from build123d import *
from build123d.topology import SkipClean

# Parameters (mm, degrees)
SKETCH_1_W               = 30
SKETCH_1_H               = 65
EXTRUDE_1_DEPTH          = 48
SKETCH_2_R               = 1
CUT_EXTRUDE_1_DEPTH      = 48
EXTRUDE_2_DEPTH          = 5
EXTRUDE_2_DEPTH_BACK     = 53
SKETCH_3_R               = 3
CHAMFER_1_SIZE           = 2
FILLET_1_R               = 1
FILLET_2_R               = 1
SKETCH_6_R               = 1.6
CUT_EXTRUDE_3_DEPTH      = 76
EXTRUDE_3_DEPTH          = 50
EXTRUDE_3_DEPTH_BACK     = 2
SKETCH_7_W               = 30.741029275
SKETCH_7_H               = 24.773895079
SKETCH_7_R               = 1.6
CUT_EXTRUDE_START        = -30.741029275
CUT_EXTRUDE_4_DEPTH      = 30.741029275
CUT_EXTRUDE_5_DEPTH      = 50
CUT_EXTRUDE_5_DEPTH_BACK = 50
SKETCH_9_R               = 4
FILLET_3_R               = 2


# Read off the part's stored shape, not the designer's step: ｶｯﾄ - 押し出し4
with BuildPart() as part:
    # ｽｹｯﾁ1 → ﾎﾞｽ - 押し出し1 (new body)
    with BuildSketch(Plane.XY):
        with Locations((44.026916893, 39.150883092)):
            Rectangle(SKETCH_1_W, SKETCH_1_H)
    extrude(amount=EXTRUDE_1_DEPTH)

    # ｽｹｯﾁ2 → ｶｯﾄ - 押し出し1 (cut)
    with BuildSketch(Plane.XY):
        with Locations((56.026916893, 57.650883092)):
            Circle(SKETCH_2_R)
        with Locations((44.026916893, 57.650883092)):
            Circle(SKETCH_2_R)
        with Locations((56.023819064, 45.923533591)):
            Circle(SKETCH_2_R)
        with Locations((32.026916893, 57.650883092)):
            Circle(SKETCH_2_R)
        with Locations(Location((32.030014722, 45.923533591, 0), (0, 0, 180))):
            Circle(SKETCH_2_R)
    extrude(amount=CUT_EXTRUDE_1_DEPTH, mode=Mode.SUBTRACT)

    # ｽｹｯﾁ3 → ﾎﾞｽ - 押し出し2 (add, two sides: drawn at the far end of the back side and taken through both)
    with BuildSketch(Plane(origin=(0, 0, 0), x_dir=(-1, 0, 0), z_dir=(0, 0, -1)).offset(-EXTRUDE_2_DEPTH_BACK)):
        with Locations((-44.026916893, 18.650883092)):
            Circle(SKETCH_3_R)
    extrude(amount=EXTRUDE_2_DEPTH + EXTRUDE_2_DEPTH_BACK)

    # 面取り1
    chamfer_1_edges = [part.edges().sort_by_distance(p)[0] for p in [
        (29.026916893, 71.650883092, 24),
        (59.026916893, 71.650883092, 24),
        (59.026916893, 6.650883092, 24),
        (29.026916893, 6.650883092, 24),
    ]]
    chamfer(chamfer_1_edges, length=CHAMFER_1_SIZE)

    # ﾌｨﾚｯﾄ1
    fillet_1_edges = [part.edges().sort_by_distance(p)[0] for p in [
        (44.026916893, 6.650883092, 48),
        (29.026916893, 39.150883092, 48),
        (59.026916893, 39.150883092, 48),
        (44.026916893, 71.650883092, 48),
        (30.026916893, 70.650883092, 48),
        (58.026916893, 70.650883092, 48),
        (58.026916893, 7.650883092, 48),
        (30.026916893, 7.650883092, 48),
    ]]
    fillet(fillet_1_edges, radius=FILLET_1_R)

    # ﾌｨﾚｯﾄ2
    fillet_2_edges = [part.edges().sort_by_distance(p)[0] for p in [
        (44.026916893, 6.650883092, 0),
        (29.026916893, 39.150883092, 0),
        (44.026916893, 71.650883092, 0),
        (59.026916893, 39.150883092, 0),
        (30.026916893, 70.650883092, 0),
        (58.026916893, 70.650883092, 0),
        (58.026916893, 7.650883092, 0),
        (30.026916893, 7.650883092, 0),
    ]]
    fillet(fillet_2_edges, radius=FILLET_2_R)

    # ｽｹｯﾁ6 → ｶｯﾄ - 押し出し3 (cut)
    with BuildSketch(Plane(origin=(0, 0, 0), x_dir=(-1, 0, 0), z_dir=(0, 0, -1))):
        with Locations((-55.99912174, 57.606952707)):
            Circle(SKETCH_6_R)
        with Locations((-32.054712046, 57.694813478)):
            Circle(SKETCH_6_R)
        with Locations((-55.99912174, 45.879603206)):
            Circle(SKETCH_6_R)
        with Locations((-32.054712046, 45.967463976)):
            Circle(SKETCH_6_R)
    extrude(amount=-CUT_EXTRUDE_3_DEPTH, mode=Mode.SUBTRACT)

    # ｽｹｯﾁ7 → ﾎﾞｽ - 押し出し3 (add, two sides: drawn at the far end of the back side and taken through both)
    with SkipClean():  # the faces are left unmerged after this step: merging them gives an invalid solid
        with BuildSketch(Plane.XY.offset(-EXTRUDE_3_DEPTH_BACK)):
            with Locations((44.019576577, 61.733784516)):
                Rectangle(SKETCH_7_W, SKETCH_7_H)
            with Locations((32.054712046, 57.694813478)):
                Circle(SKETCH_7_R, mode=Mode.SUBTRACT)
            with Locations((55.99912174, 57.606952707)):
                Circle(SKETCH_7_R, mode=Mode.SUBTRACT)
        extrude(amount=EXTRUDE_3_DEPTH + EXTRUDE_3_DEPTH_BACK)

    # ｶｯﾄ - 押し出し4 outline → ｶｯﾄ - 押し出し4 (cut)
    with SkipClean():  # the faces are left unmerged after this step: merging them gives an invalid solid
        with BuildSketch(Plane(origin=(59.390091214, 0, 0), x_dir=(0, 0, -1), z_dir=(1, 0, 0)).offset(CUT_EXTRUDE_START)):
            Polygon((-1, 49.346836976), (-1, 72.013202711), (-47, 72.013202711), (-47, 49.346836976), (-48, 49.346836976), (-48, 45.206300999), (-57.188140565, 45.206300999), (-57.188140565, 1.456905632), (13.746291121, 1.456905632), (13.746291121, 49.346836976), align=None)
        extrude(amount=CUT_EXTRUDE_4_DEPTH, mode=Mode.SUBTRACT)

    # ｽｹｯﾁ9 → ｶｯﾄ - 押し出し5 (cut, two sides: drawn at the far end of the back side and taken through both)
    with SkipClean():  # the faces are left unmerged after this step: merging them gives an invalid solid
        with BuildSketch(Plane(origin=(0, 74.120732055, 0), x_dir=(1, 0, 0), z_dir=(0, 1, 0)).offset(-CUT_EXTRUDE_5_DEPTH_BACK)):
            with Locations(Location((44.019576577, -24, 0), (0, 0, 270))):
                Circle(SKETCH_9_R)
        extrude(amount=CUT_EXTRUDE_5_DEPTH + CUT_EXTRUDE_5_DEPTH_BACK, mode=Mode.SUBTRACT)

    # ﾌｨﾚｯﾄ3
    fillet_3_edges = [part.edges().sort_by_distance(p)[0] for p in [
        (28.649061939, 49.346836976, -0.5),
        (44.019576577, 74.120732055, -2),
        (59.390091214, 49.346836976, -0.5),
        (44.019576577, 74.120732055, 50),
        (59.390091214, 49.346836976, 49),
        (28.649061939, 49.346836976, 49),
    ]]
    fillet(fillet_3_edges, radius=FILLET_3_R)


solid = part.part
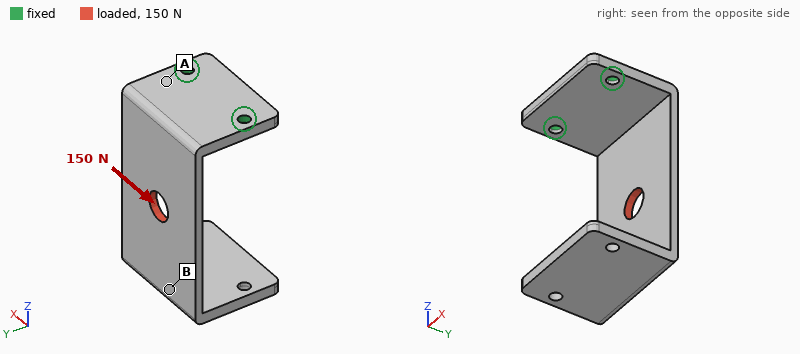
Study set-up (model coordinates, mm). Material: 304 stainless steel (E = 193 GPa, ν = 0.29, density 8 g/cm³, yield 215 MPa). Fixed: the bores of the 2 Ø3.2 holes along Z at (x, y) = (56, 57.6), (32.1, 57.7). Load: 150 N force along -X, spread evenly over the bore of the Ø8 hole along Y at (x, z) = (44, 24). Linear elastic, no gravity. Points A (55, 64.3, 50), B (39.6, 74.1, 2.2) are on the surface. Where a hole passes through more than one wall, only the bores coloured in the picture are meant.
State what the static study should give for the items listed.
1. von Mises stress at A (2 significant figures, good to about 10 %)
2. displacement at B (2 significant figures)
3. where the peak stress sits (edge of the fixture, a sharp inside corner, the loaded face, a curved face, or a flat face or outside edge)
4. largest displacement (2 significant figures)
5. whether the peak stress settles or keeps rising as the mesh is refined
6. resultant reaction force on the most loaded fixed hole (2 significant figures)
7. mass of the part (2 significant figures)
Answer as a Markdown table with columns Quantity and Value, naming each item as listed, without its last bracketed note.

| Quantity | Value |
|---|---|
| von Mises stress at A | 42 MPa |
| displacement at B | 66 µm |
| where the peak stress sits | edge of the fixture |
| largest displacement | 95 µm |
| whether the peak stress settles or keeps rising as the mesh is refined | keeps rising |
| resultant reaction force on the most loaded fixed hole | 190 N |
| mass of the part | 58 g |
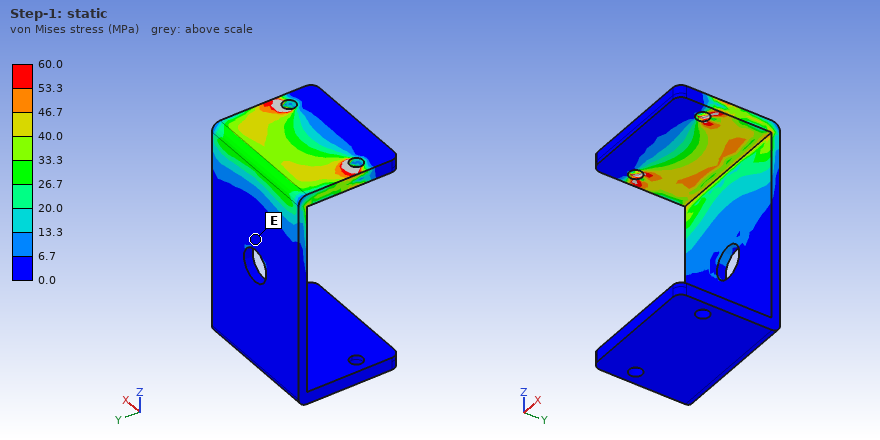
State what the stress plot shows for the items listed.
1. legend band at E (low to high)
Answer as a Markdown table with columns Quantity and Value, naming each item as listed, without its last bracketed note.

| Quantity | Value |
|---|---|
| legend band at E | 0.0 to 6.7 MPa |
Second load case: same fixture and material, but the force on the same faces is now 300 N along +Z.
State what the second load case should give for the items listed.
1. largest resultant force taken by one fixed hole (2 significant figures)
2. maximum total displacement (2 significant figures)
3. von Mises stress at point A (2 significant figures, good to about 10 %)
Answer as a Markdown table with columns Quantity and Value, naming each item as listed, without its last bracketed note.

| Quantity | Value |
|---|---|
| largest resultant force taken by one fixed hole | 150 N |
| maximum total displacement | 0.17 mm |
| von Mises stress at point A | 60 MPa |
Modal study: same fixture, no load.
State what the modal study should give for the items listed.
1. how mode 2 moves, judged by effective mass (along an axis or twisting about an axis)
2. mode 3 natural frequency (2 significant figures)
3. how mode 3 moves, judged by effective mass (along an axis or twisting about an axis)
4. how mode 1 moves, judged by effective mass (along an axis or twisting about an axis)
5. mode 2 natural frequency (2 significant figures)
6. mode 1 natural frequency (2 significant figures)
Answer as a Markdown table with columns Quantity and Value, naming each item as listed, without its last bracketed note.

| Quantity | Value |
|---|---|
| how mode 2 moves, judged by effective mass | along X |
| mode 3 natural frequency | 1300 Hz |
| how mode 3 moves, judged by effective mass | along Z |
| how mode 1 moves, judged by effective mass | along Y |
| mode 2 natural frequency | 720 Hz |
| mode 1 natural frequency | 300 Hz |
